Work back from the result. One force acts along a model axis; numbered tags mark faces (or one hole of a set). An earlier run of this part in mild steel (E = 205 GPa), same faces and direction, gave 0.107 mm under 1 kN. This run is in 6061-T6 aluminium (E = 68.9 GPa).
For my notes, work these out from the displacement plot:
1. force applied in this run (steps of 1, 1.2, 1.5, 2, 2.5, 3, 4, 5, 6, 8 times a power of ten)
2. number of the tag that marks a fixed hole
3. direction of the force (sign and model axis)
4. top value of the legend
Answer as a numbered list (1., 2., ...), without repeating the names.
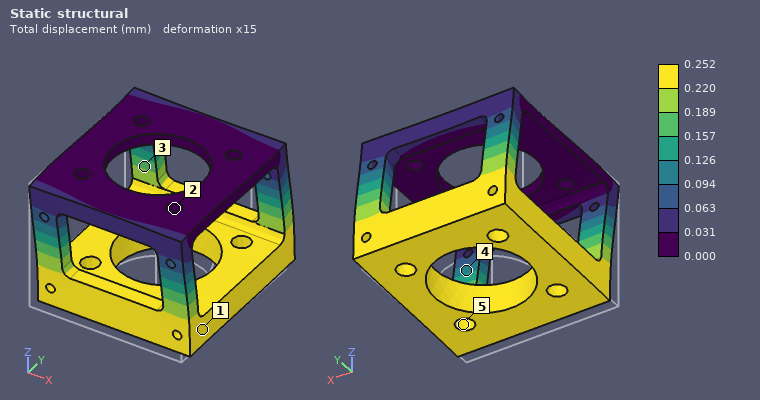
1. 800 N
2. 2
3. +Y
4. 0.252 mm
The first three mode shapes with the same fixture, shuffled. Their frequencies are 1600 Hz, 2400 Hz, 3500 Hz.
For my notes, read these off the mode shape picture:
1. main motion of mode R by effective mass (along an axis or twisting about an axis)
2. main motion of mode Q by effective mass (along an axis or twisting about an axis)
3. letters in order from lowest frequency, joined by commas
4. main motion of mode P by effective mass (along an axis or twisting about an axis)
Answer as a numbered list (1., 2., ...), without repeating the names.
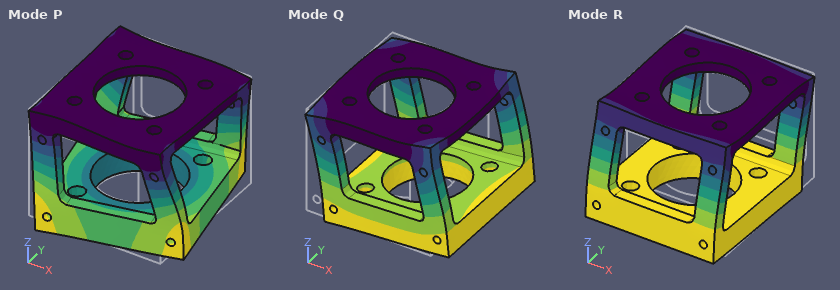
1. along Y
2. along X
3. R, Q, P
4. twisting about Z
